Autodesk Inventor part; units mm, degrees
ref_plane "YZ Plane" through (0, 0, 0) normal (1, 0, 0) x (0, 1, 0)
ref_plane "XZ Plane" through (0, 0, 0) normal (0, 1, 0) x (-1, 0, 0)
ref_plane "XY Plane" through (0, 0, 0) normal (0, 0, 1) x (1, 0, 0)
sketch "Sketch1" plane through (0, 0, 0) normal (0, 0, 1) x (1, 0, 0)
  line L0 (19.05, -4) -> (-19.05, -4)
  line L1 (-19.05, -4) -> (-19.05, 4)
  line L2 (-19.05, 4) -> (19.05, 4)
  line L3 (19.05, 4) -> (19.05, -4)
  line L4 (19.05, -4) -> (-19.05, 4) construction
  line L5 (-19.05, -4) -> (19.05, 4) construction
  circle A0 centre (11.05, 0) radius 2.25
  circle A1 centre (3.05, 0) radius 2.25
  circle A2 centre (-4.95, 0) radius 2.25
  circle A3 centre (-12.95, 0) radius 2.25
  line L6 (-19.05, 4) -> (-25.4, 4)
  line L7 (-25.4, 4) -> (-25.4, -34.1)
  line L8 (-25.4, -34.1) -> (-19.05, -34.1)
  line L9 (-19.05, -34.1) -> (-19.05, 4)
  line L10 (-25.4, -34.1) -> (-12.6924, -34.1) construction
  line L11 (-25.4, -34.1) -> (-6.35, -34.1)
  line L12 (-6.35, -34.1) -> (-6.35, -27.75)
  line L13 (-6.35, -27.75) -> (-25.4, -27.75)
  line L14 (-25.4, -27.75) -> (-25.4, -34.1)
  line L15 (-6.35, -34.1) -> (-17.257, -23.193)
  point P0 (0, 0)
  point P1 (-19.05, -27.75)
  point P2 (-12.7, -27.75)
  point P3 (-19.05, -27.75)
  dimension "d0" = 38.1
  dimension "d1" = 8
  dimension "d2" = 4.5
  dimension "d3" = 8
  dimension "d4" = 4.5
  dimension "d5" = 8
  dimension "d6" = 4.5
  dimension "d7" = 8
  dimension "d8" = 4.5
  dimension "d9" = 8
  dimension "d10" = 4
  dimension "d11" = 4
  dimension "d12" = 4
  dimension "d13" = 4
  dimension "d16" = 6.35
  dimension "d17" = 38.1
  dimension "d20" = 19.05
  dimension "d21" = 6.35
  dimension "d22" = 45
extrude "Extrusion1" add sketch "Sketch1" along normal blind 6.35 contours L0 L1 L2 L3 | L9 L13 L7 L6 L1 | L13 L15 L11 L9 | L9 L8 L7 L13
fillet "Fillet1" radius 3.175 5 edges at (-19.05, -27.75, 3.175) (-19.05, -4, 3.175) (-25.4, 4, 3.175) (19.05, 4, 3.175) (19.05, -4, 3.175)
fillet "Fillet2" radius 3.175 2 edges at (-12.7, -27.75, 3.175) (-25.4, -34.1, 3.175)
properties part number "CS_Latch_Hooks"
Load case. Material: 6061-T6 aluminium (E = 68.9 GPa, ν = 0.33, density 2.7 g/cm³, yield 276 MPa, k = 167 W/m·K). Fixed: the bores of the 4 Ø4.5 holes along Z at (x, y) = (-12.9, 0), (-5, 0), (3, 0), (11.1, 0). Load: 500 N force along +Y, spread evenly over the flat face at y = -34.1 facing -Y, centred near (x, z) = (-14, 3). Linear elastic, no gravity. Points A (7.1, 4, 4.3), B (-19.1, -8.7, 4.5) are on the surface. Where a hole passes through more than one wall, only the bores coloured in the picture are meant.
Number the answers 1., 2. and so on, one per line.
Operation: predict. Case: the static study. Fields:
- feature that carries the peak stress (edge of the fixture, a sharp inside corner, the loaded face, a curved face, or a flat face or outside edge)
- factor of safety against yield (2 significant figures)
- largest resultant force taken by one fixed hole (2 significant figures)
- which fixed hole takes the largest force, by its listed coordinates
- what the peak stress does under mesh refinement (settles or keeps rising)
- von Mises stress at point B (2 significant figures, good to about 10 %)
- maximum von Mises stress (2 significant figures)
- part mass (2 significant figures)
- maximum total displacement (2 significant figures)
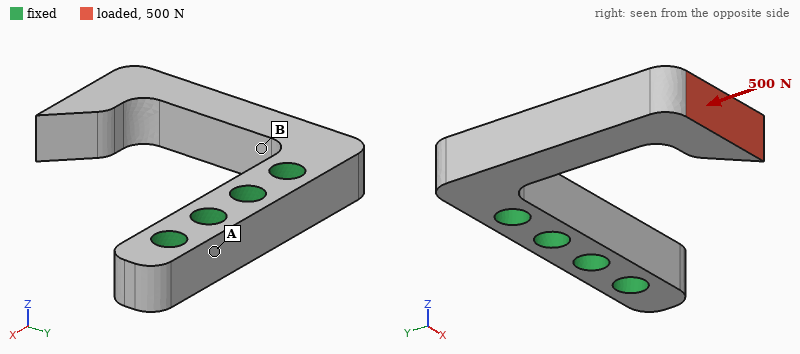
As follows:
1. a curved face
2. 2.0
3. 500 N
4. (-12.9, 0)
5. settles
6. 110 MPa
7. 140 MPa
8. 9.2 g
9. 0.29 mm
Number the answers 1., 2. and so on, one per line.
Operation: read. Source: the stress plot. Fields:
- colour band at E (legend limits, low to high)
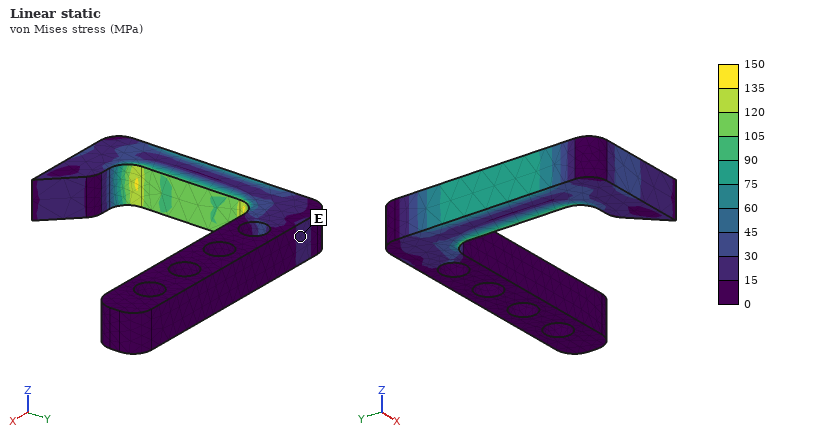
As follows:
1. 15 to 30 MPa
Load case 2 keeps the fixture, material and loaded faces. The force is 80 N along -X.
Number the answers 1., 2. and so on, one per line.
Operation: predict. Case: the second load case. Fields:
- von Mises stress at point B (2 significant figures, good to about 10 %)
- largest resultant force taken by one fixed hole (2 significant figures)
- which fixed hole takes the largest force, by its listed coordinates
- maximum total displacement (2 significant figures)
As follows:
1. 48 MPa
2. 89 N
3. (-12.9, 0)
4. 0.15 mm
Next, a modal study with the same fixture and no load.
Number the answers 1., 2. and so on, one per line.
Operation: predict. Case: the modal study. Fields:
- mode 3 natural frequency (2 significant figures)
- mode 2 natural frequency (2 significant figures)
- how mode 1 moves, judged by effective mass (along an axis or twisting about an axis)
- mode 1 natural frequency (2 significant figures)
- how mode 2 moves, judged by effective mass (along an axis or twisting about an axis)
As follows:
1. 9000 Hz
2. 3000 Hz
3. along Z
4. 2700 Hz
5. along X
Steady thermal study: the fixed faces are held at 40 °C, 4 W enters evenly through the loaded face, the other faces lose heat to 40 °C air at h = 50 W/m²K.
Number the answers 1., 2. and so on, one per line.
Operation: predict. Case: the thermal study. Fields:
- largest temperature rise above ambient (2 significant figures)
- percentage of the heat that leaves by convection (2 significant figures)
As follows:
1. 21 K
2. 15 %
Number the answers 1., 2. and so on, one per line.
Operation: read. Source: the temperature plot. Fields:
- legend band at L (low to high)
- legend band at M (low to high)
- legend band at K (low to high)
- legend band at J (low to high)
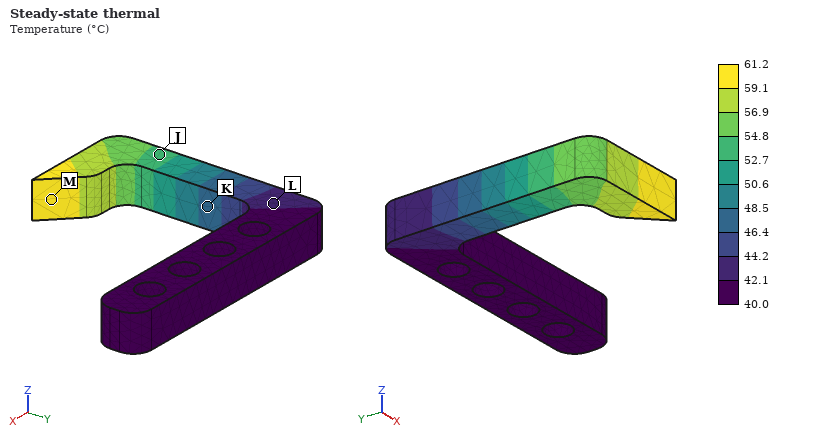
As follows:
1. 42.1 to 44.2 °C
2. 59.1 to 61.2 °C
3. 46.4 to 48.5 °C
4. 52.7 to 54.8 °C
